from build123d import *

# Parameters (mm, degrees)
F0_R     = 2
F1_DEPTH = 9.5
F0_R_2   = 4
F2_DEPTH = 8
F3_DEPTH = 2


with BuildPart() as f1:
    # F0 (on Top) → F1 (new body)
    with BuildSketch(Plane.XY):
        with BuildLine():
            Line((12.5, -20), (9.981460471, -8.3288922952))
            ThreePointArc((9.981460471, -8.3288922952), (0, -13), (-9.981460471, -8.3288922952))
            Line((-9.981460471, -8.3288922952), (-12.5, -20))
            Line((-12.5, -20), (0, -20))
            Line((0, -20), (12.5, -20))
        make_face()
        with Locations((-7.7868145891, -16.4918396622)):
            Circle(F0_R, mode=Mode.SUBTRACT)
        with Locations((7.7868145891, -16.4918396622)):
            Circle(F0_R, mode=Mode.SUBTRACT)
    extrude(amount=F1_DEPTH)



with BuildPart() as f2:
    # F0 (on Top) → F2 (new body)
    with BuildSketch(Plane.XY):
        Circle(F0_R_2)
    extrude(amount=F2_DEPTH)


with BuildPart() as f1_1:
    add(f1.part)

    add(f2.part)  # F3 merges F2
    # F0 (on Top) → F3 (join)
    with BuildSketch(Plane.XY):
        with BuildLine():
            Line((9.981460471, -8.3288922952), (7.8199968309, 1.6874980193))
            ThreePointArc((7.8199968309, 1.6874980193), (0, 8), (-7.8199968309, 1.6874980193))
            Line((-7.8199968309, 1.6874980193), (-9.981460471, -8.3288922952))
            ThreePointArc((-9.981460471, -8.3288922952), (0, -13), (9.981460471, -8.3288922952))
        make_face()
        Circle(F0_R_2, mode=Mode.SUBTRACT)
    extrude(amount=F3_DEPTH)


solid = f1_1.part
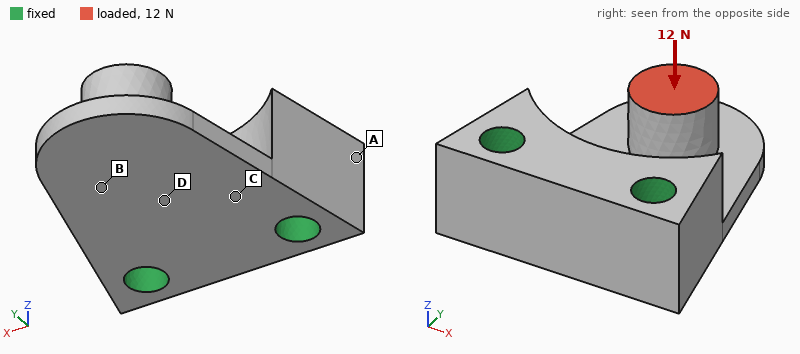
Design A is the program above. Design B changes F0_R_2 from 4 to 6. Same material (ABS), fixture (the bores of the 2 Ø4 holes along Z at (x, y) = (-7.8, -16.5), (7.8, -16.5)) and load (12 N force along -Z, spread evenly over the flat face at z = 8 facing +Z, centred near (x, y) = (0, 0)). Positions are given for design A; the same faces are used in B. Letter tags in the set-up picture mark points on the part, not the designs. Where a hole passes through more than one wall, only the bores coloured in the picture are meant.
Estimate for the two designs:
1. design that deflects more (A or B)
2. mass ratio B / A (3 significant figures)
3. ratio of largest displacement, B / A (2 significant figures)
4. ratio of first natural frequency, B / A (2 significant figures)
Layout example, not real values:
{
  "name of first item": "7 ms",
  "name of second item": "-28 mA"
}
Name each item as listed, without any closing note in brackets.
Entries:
{
  "design that deflects more": "A",
  "mass ratio B / A": "1.15",
  "ratio of largest displacement, B / A": "0.88",
  "ratio of first natural frequency, B / A": "0.84"
}
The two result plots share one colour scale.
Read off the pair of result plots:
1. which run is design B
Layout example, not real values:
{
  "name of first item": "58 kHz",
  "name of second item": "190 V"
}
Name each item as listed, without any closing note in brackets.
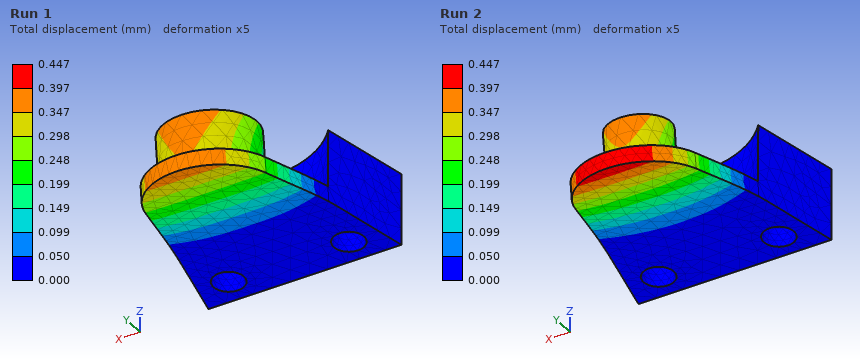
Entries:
{
  "which run is design B": "Run 1"
}
